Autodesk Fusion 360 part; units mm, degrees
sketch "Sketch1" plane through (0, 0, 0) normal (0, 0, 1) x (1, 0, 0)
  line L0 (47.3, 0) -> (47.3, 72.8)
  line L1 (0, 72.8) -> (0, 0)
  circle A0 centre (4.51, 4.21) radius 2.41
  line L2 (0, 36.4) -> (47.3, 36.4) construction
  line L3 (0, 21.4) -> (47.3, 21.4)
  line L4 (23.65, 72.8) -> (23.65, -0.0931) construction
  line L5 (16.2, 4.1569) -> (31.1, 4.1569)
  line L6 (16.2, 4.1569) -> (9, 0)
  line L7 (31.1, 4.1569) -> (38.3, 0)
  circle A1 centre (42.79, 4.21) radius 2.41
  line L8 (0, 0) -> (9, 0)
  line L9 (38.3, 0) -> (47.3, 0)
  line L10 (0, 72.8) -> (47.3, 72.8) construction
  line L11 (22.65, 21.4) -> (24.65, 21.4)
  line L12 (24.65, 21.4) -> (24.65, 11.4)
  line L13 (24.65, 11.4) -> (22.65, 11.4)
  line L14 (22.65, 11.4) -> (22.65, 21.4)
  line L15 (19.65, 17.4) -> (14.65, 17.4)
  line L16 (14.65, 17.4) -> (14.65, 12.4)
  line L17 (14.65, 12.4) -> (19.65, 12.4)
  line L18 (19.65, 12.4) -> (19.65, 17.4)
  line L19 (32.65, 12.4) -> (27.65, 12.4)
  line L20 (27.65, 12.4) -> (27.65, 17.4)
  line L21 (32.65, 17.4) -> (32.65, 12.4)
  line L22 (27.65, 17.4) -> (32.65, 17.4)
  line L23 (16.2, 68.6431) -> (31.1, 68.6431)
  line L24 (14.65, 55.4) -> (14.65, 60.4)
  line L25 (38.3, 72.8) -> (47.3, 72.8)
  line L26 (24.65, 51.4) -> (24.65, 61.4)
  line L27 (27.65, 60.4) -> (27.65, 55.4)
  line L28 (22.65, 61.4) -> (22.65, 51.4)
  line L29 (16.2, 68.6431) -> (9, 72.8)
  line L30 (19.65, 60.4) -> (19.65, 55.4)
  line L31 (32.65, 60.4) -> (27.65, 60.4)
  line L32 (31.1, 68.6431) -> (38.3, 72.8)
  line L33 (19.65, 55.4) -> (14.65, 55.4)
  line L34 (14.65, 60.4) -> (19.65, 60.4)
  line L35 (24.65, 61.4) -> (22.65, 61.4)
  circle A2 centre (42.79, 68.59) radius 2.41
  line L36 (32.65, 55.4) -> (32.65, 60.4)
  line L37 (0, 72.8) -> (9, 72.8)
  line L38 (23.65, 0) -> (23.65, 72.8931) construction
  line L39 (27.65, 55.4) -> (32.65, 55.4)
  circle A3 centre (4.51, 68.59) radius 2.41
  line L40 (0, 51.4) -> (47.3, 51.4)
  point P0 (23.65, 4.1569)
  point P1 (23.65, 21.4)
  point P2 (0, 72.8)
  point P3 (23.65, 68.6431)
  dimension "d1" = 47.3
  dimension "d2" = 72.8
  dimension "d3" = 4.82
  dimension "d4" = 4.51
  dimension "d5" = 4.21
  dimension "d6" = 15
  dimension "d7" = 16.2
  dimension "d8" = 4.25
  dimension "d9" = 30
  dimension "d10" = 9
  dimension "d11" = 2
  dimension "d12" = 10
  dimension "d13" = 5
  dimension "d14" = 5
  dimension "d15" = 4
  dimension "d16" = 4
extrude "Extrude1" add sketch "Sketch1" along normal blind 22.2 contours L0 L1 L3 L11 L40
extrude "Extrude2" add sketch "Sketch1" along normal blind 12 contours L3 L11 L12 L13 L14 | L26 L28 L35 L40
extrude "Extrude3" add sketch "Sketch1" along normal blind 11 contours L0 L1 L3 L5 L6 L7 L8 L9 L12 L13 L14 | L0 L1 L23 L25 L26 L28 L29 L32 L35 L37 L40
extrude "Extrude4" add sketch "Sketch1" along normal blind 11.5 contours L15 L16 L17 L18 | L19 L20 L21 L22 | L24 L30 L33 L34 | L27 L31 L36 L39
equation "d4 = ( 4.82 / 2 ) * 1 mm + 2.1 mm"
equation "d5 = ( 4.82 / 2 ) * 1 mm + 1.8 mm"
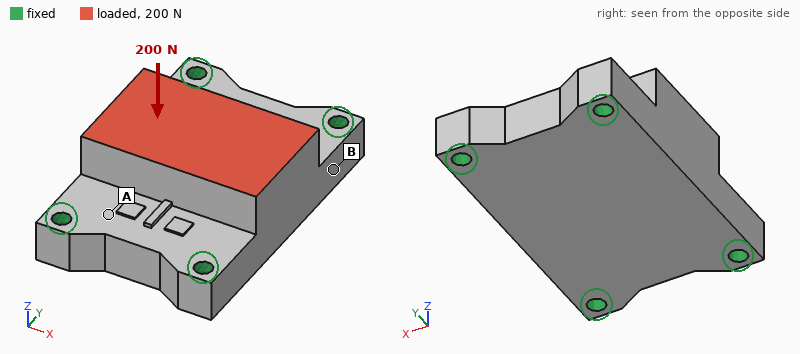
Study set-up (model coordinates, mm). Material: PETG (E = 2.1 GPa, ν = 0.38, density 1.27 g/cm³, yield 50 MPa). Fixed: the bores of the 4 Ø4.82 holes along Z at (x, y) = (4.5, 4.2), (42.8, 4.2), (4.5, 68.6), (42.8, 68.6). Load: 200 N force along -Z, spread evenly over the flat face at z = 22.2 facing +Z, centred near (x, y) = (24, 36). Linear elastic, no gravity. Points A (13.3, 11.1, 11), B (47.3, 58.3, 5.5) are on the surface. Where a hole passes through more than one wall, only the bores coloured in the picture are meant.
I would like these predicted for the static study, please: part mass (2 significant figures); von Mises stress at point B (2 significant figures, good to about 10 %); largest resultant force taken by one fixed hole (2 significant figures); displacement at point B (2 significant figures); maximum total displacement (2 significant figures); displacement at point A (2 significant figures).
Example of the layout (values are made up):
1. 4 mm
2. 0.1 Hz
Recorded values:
1. 65 g
2. 0.92 MPa
3. 53 N
4. 8.1 µm
5. 20 µm
6. 8.1 µm
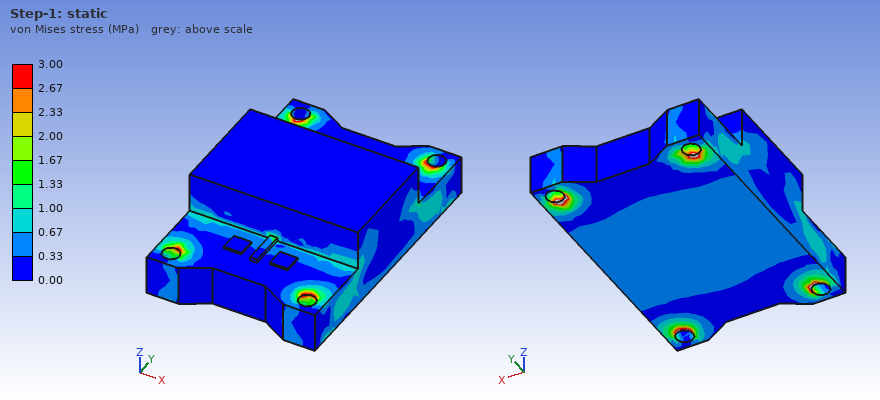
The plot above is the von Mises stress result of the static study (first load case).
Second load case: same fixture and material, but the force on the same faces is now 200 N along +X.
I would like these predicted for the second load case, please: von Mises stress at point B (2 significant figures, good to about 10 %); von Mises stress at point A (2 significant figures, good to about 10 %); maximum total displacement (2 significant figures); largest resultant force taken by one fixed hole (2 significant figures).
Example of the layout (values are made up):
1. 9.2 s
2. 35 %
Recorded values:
1. 1.3 MPa
2. 0.93 MPa
3. 36 µm
4. 81 N
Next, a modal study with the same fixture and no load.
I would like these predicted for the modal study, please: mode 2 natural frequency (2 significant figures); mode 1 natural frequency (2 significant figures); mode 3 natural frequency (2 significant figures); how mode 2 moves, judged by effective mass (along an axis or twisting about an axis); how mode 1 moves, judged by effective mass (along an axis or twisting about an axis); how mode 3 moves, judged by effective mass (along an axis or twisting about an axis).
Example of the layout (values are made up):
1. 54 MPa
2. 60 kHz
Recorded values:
1. 2700 Hz
2. 2400 Hz
3. 4200 Hz
4. along X
5. along Z
6. along X
